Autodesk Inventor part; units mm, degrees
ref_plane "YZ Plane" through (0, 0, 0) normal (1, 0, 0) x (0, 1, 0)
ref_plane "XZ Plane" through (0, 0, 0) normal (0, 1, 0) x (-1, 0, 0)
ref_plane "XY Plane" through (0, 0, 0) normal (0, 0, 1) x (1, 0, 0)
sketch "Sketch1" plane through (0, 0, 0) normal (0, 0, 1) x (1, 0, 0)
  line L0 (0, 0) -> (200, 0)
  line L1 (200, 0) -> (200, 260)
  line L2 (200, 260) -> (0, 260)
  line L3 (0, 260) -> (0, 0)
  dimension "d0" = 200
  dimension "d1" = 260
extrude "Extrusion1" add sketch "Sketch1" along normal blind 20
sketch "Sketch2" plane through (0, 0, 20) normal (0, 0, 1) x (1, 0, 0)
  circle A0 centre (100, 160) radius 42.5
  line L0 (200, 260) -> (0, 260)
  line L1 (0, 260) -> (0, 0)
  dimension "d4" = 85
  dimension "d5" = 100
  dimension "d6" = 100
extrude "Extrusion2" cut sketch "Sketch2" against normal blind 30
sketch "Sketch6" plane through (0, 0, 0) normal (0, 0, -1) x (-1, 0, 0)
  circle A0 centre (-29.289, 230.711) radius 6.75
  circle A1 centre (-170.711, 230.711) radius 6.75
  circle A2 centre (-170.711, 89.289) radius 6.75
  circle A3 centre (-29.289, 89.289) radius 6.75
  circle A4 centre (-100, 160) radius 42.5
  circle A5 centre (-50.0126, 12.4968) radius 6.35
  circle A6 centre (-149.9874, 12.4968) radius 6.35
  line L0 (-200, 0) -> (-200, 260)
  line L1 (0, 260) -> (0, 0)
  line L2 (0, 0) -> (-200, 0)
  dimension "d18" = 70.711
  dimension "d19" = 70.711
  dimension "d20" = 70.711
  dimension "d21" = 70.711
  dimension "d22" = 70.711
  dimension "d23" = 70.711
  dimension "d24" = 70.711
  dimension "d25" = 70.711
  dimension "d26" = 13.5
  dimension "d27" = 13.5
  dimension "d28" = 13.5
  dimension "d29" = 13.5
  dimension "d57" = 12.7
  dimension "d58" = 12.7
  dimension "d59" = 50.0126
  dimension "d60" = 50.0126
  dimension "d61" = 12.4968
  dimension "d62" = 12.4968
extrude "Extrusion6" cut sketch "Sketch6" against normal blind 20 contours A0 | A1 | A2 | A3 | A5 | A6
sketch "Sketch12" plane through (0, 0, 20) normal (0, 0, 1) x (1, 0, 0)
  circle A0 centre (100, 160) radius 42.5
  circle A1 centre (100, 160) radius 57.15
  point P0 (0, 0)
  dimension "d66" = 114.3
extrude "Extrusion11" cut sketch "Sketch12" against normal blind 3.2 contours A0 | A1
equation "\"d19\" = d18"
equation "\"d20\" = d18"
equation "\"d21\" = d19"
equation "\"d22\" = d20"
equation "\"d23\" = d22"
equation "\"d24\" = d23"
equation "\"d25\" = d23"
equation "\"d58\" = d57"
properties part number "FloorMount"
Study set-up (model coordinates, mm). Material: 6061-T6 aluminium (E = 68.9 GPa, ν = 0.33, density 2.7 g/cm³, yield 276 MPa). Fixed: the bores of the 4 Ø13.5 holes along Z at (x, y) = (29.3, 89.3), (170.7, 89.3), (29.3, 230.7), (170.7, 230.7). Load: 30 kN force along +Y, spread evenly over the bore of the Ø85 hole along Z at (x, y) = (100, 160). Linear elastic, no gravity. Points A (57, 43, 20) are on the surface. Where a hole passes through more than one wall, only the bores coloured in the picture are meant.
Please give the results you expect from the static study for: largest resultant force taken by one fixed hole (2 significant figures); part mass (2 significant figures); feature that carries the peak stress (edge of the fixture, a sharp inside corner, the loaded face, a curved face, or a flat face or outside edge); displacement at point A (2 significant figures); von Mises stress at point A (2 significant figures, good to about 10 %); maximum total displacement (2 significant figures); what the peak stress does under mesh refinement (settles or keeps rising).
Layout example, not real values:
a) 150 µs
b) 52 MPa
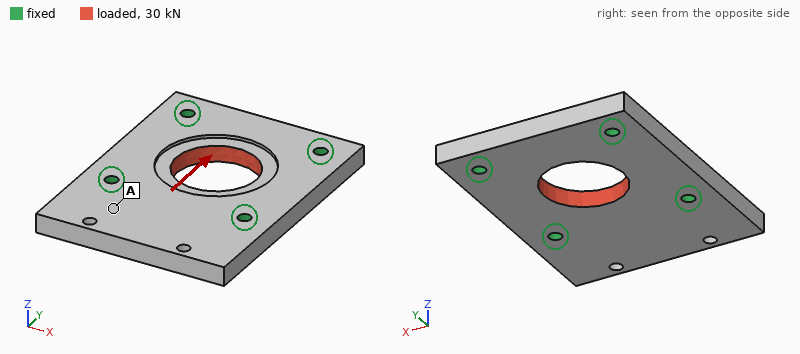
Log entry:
a) 7.9 kN
b) 2.4 kg
c) edge of the fixture
d) 3.5 µm
e) 2.5 MPa
f) 15 µm
g) keeps rising
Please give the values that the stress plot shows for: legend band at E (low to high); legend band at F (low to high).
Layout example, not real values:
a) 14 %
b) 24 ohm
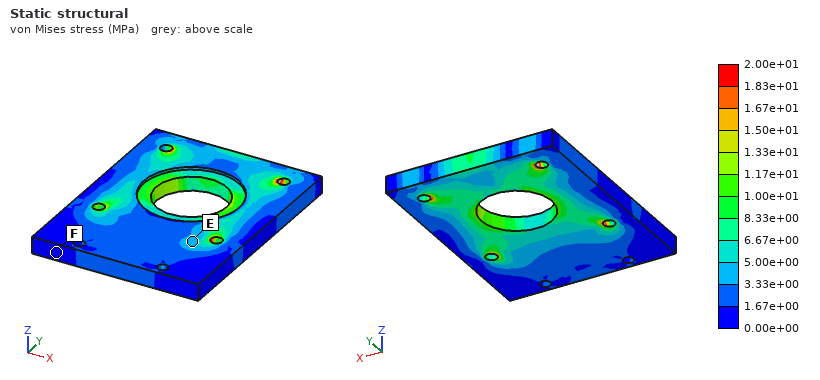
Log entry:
a) 3.33e+00 to 5.00e+00 MPa
b) 0.00e+00 to 1.67e+00 MPa
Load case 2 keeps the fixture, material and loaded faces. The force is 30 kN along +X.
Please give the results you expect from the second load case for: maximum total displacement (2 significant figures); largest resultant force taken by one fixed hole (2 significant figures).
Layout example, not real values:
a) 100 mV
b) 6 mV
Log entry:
a) 14 µm
b) 7.9 kN
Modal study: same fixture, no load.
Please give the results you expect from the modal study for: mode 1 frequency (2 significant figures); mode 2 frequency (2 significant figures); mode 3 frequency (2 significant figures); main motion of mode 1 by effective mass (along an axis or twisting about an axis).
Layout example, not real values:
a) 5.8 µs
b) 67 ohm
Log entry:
a) 1700 Hz
b) 2700 Hz
c) 3900 Hz
d) along Z
